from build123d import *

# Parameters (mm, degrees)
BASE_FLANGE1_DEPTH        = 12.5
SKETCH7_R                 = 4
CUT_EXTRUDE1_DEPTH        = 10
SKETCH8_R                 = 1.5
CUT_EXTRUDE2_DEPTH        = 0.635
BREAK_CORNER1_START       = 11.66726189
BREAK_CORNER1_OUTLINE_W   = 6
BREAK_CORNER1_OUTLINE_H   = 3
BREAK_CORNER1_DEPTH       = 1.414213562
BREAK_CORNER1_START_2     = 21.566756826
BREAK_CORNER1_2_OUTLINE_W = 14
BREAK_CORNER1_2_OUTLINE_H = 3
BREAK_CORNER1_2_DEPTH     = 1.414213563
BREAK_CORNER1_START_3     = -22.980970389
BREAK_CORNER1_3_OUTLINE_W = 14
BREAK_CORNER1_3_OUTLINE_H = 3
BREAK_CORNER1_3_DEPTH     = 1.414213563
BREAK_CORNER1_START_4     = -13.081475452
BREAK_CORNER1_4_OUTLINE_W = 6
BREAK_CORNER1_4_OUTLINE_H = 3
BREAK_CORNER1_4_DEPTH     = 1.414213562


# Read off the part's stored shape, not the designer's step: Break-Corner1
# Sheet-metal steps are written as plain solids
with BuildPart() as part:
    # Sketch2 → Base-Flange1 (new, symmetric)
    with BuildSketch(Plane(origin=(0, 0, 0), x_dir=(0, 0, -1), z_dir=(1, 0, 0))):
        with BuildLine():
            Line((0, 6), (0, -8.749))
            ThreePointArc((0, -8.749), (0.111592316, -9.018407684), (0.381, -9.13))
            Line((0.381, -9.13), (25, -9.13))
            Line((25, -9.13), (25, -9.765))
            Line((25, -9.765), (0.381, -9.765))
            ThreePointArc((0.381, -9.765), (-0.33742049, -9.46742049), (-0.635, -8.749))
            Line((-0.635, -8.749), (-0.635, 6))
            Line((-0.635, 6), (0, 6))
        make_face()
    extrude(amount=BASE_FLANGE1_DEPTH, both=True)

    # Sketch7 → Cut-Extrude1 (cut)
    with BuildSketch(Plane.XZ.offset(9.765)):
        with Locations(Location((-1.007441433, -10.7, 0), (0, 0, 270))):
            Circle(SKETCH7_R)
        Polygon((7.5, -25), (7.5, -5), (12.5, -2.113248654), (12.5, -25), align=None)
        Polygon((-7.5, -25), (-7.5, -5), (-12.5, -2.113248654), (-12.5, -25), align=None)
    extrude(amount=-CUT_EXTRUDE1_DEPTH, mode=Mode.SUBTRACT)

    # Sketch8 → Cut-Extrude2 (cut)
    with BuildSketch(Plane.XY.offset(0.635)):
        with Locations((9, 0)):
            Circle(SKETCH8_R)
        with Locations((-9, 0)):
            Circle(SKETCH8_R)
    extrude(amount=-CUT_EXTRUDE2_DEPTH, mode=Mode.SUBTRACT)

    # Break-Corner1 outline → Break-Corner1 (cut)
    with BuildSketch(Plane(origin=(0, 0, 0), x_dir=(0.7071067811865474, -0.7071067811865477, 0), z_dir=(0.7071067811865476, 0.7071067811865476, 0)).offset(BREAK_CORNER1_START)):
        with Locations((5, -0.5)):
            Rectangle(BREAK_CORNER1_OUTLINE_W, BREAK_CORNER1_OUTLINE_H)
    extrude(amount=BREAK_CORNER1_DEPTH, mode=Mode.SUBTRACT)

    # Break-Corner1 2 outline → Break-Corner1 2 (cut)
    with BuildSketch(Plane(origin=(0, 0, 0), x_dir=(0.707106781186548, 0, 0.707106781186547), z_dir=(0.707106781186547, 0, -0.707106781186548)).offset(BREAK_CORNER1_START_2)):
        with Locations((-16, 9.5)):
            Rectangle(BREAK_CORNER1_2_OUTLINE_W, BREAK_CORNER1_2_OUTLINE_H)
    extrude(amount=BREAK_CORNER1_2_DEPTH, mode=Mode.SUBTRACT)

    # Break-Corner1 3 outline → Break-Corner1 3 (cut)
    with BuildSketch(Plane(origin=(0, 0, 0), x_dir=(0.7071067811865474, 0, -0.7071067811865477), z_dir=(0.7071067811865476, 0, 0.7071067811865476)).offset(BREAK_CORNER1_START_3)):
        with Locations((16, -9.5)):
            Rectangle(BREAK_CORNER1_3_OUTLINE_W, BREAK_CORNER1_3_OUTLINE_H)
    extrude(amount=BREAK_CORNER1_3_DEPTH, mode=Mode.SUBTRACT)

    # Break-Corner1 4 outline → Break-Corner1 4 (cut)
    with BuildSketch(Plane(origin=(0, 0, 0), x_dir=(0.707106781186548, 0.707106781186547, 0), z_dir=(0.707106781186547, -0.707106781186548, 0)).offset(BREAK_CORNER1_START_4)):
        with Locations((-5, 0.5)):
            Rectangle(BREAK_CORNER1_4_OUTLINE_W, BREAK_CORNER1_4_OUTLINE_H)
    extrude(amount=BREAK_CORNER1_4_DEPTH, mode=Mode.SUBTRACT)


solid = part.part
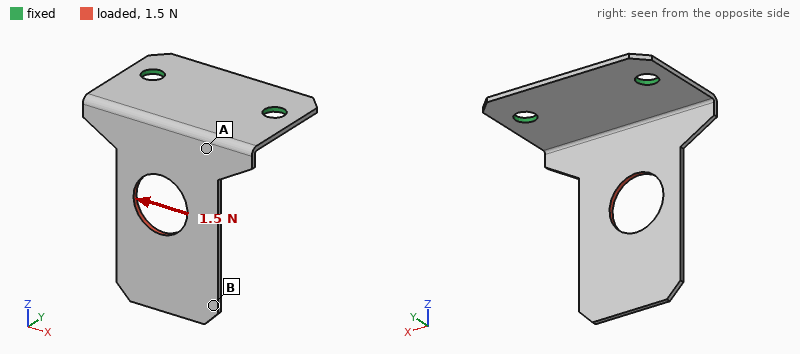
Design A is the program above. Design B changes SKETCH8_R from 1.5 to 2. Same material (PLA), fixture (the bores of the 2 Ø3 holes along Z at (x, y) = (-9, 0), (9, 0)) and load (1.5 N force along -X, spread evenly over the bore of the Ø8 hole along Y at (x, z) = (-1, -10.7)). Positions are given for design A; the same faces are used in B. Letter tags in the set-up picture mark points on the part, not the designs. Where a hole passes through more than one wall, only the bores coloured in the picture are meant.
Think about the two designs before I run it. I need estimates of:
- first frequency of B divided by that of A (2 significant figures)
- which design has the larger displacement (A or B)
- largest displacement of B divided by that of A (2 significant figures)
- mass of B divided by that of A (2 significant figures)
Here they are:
1.0
A
0.86
0.98
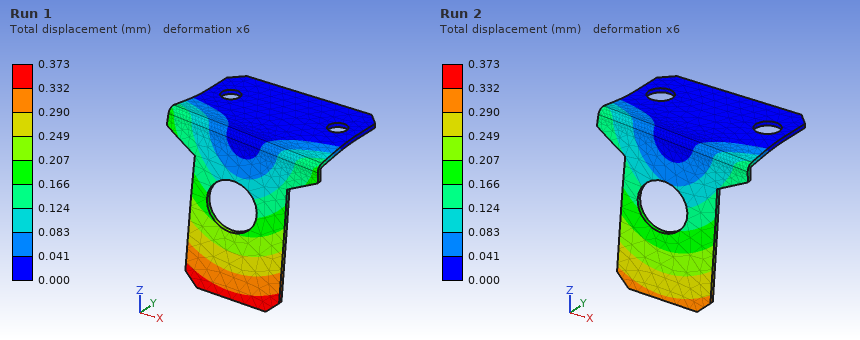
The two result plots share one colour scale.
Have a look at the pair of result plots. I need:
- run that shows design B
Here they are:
Run 2
